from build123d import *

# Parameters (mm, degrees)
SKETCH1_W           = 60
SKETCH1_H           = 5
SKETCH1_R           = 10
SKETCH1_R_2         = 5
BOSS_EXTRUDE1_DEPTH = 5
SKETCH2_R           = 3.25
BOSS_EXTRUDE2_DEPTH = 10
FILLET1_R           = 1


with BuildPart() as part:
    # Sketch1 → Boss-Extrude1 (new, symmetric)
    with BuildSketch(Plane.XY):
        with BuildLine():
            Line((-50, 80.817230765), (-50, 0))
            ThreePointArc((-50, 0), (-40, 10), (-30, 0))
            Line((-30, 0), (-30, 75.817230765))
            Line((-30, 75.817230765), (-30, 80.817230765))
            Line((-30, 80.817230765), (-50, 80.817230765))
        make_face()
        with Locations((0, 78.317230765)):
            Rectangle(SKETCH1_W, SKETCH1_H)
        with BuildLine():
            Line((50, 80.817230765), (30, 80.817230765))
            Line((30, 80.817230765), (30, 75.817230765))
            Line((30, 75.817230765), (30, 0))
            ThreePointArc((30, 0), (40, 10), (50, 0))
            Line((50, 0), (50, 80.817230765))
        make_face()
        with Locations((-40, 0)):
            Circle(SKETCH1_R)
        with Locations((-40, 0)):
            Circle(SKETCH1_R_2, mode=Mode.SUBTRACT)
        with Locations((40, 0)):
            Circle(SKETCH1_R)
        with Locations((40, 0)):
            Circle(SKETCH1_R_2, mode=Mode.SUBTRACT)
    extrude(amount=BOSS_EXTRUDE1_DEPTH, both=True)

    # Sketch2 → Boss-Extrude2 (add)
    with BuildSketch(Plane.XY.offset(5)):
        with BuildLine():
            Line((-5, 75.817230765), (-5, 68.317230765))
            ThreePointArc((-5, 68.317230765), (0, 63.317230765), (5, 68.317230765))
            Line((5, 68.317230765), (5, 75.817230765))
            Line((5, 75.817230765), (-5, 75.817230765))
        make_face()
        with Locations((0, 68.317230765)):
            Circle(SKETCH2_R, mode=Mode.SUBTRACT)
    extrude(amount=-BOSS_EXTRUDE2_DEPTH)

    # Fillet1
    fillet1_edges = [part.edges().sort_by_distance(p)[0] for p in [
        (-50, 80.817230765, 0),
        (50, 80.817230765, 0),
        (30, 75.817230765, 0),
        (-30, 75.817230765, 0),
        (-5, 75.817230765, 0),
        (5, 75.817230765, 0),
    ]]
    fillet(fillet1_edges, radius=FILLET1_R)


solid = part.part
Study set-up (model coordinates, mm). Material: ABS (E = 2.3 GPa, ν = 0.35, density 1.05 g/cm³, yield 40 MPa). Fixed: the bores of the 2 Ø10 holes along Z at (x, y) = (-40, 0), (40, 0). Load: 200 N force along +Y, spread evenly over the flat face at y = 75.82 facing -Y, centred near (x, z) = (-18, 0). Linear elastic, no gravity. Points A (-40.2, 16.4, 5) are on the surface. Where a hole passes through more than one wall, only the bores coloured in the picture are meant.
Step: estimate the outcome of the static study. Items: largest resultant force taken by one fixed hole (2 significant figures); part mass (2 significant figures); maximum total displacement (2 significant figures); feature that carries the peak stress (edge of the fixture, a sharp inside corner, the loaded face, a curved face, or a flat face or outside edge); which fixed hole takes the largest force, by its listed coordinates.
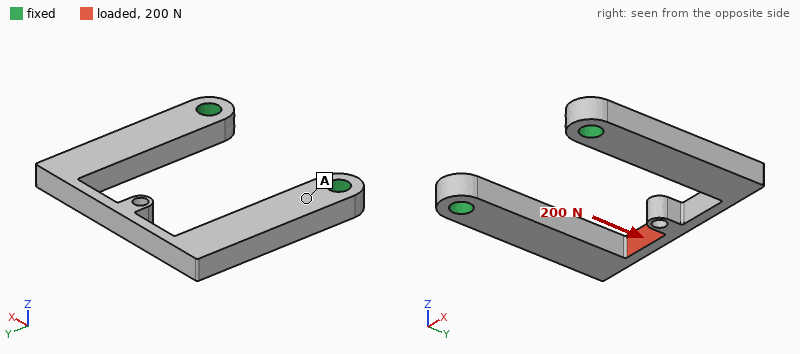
170 N
40 g
0.72 mm
a curved face
(-40, 0)
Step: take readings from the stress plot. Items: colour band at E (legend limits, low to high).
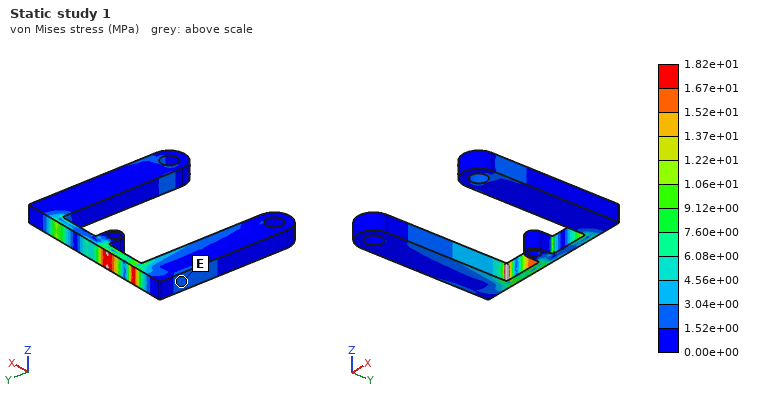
1.52e+00 to 3.04e+00 MPa
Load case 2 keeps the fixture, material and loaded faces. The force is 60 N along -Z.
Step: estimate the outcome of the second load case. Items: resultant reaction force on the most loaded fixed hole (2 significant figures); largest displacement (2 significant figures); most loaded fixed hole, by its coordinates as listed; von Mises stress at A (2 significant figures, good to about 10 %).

39 N
1.4 mm
(-40, 0)
6.8 MPa
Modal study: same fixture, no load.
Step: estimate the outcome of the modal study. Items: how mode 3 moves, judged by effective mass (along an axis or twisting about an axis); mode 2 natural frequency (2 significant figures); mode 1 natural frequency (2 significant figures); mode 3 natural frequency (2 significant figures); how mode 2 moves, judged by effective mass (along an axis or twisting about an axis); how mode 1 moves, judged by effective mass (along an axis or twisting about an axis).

along X
510 Hz
330 Hz
590 Hz
twisting about Y
along Z
